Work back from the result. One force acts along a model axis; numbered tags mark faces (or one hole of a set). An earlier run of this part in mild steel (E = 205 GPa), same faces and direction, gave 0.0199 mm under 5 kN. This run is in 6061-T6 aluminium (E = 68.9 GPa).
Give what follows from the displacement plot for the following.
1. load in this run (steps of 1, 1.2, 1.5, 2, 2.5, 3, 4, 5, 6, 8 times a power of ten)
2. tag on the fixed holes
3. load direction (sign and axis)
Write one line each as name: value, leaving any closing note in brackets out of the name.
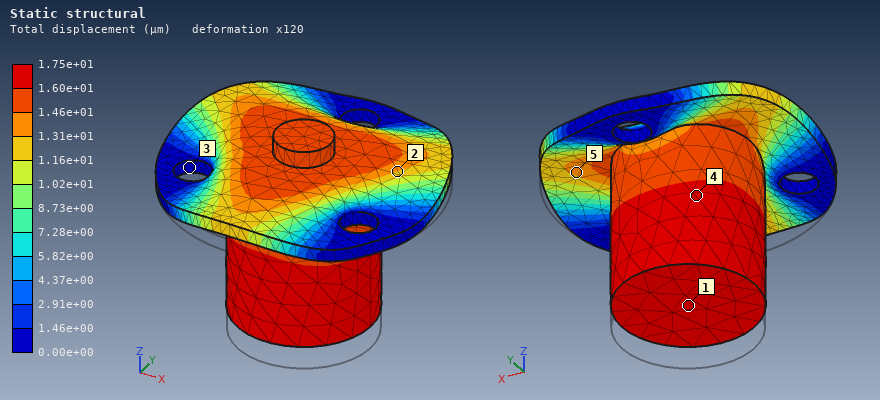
load in this run: 1.5 kN
tag on the fixed holes: 3
load direction: +Z
